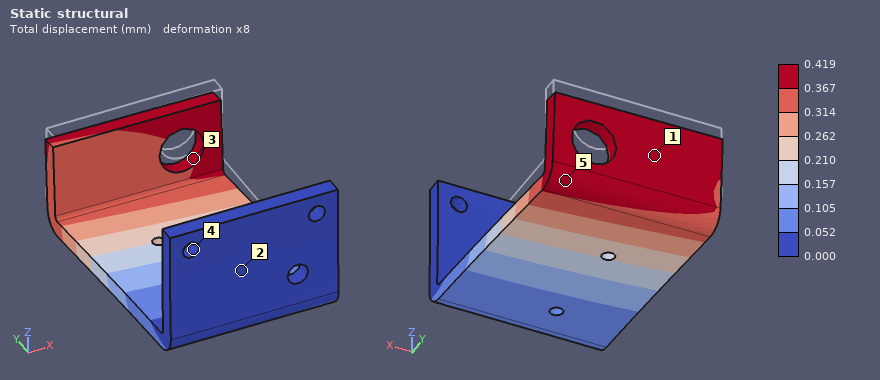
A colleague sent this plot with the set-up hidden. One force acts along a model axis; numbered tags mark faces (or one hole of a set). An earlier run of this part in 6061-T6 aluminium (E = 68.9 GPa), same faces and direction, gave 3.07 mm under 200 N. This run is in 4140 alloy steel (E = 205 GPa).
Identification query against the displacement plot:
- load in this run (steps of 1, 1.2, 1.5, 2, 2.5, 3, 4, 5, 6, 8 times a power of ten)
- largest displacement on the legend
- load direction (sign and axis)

80 N
0.419 mm
-Z
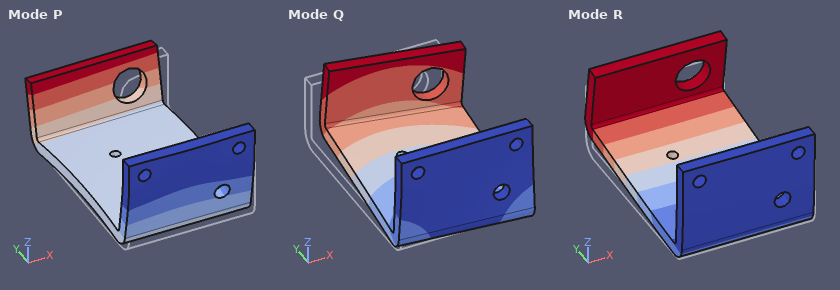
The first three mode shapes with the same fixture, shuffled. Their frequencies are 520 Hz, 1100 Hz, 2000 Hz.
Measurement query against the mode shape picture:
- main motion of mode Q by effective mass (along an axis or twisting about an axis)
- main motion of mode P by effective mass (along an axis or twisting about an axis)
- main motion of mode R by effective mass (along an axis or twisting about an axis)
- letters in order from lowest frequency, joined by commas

along X
along Y
along Z
R, Q, P
